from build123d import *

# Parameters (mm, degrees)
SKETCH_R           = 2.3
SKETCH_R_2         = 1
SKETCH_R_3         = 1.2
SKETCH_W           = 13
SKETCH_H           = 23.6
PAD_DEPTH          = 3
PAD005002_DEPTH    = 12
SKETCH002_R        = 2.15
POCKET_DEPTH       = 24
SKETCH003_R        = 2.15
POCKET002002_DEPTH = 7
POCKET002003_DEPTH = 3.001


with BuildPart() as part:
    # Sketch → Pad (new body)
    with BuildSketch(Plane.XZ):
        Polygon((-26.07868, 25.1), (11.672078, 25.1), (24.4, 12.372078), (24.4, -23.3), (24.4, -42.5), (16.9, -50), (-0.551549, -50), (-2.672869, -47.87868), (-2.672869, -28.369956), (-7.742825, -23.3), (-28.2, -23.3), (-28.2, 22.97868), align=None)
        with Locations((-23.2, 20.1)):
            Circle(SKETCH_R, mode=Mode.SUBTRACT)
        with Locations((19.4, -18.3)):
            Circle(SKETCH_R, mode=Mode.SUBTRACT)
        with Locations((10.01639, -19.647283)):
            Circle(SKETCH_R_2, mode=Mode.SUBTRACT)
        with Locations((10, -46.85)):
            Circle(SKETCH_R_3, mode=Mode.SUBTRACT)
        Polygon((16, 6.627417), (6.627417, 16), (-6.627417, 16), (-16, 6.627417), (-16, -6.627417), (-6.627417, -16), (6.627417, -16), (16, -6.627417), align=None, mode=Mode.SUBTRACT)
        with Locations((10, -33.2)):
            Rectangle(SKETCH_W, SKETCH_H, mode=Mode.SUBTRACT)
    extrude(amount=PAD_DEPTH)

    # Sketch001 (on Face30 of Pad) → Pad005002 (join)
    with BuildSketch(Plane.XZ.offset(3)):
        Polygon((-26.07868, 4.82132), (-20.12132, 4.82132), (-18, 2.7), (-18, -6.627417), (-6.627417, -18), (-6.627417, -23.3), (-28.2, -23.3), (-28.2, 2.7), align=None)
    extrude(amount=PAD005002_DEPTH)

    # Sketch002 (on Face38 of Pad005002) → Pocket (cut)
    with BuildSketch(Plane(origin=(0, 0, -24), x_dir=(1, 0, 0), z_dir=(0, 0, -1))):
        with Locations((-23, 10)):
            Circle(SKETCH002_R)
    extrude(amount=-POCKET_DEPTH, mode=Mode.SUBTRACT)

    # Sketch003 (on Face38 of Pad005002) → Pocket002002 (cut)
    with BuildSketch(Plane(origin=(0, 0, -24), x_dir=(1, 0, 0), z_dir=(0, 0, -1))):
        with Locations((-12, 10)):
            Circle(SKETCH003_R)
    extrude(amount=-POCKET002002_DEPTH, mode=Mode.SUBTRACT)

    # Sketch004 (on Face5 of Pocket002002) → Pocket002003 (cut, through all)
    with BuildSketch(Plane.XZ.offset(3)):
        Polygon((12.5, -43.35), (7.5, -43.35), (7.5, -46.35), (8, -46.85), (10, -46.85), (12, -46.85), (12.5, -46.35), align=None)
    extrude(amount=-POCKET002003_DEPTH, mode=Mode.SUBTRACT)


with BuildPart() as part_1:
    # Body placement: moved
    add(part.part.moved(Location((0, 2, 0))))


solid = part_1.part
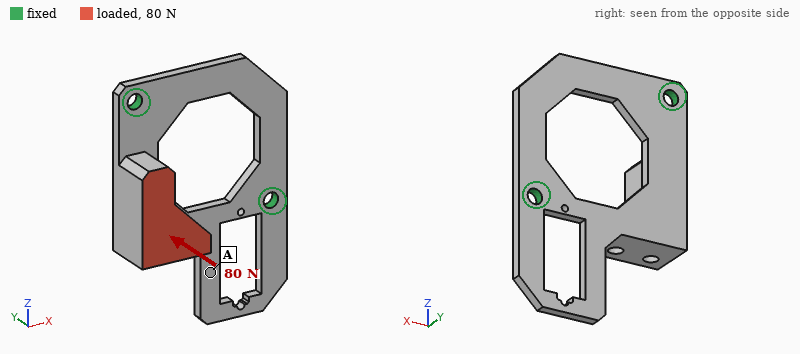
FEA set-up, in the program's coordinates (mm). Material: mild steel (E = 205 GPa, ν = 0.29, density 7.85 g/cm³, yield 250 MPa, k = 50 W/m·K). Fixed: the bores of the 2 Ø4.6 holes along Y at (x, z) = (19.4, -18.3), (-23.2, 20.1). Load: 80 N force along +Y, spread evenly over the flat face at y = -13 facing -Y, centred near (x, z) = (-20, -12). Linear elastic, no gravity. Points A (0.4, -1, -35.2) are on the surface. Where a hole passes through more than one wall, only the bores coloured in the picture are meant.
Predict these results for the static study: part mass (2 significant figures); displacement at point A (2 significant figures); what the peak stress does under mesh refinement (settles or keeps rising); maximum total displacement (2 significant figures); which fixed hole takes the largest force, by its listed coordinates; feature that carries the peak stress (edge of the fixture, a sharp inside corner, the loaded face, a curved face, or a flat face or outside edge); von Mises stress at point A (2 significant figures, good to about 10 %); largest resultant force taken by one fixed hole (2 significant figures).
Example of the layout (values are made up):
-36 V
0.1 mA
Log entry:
81 g
26 µm
keeps rising
53 µm
(-23.2, 20.1)
edge of the fixture
6.7 MPa
47 N
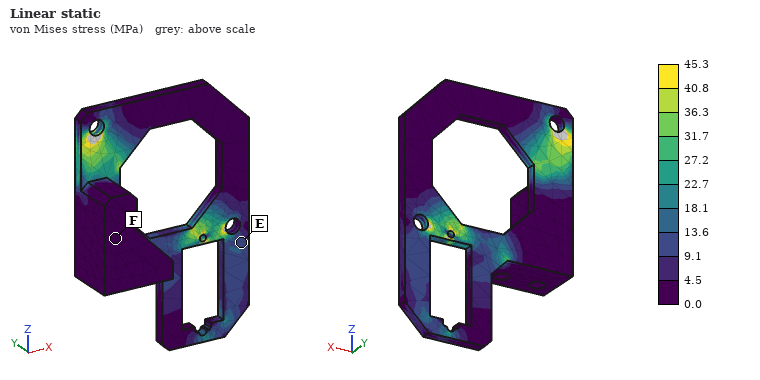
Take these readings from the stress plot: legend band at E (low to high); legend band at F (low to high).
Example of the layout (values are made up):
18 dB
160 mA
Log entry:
9.1 to 13.6 MPa
0.0 to 4.5 MPa
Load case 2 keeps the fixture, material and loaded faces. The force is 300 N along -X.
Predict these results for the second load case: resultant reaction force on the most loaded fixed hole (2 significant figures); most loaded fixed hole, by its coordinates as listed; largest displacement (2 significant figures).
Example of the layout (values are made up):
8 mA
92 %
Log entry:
200 N
(19.4, -18.3)
0.12 mm
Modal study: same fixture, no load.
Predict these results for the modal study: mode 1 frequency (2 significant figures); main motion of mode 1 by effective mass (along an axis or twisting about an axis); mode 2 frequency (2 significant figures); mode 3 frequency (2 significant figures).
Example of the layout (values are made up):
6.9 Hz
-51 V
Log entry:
1100 Hz
along Y
2500 Hz
2600 Hz
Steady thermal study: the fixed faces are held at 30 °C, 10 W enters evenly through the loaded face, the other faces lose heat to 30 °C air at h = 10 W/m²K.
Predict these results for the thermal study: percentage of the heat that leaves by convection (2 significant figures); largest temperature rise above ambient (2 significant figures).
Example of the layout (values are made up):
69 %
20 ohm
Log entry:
18 %
64 K
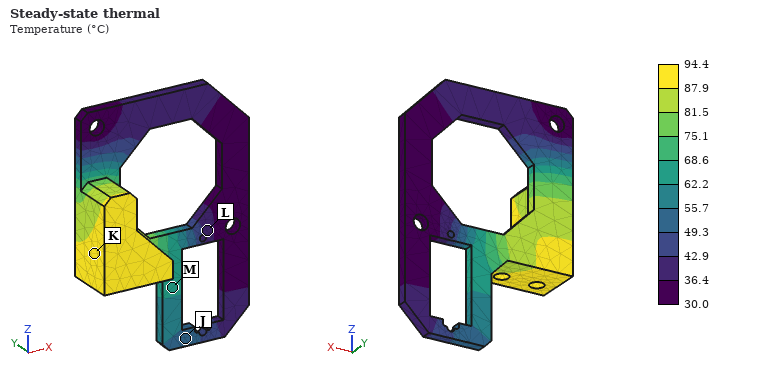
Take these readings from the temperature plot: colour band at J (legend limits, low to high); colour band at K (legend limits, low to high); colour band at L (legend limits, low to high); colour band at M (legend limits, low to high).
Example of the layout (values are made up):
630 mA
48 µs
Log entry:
49.3 to 55.7 °C
87.9 to 94.4 °C
36.4 to 42.9 °C
62.2 to 68.6 °C
